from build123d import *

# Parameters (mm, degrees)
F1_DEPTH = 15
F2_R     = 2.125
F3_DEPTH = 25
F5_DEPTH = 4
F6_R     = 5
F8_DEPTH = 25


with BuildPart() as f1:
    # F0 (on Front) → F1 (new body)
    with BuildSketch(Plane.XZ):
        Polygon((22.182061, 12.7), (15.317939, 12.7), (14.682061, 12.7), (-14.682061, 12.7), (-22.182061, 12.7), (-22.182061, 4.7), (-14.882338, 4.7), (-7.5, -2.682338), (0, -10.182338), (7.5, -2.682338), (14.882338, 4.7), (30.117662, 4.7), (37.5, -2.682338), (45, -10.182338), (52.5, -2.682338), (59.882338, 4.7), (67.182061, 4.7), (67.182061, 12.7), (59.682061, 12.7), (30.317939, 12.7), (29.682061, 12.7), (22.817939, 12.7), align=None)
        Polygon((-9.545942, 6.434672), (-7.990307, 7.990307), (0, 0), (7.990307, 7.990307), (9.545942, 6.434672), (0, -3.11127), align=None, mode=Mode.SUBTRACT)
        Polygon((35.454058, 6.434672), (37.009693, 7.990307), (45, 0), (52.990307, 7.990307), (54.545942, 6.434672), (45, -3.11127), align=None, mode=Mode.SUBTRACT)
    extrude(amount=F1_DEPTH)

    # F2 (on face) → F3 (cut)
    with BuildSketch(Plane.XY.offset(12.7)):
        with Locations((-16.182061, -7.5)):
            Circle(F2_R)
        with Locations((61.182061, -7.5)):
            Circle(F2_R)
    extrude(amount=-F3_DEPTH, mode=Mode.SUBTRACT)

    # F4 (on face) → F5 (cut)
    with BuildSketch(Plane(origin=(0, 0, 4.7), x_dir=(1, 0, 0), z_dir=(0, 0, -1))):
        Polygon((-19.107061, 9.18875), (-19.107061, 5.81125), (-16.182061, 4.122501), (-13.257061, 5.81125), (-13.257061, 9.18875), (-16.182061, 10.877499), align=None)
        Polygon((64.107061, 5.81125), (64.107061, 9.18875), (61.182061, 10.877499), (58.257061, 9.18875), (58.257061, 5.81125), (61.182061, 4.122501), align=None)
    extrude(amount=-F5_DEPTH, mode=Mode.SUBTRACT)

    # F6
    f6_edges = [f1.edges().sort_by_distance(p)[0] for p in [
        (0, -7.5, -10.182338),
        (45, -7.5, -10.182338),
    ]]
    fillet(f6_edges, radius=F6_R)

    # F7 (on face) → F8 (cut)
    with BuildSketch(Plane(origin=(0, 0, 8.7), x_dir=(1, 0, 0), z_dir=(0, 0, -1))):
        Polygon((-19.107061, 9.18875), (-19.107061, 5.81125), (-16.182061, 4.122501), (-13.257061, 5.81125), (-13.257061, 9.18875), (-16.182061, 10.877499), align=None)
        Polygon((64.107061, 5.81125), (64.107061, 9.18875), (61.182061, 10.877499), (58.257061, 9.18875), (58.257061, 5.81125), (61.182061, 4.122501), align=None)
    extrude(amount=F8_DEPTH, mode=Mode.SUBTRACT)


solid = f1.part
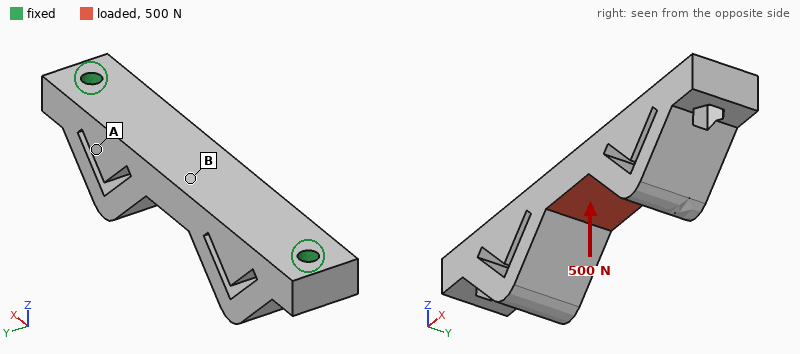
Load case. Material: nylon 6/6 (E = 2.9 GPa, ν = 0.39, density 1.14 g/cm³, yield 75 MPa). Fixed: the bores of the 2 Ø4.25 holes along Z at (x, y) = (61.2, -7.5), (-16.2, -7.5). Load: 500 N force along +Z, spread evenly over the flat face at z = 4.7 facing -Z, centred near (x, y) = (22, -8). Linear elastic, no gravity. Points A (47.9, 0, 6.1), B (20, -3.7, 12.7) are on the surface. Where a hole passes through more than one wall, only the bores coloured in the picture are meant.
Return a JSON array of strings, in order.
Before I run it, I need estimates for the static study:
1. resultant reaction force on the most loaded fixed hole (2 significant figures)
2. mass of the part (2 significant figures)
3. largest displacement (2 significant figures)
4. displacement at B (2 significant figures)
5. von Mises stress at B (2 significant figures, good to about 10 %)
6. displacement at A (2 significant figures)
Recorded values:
["390 N", "17 g", "1.1 mm", "1.0 mm", "25 MPa", "0.40 mm"]
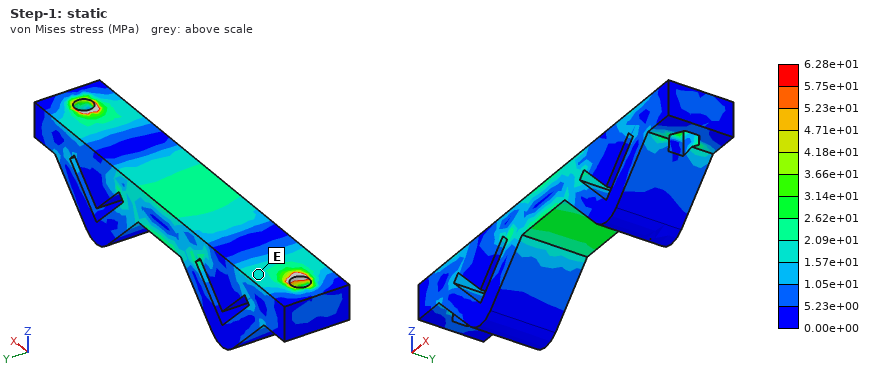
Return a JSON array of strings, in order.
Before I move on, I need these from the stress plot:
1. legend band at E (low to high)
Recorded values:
["1.57e+01 to 2.09e+01 MPa"]
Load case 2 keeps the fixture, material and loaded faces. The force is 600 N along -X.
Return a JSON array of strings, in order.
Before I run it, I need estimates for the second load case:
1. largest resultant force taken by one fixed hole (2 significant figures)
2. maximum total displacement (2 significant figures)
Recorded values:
["300 N", "59 µm"]
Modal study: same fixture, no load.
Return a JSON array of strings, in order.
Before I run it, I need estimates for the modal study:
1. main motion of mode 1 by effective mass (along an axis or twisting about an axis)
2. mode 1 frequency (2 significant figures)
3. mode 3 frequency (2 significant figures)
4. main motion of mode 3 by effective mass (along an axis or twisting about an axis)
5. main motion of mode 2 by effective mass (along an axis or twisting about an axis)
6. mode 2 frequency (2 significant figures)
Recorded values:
["along Z", "1300 Hz", "3000 Hz", "twisting about X", "along Y", "1800 Hz"]
